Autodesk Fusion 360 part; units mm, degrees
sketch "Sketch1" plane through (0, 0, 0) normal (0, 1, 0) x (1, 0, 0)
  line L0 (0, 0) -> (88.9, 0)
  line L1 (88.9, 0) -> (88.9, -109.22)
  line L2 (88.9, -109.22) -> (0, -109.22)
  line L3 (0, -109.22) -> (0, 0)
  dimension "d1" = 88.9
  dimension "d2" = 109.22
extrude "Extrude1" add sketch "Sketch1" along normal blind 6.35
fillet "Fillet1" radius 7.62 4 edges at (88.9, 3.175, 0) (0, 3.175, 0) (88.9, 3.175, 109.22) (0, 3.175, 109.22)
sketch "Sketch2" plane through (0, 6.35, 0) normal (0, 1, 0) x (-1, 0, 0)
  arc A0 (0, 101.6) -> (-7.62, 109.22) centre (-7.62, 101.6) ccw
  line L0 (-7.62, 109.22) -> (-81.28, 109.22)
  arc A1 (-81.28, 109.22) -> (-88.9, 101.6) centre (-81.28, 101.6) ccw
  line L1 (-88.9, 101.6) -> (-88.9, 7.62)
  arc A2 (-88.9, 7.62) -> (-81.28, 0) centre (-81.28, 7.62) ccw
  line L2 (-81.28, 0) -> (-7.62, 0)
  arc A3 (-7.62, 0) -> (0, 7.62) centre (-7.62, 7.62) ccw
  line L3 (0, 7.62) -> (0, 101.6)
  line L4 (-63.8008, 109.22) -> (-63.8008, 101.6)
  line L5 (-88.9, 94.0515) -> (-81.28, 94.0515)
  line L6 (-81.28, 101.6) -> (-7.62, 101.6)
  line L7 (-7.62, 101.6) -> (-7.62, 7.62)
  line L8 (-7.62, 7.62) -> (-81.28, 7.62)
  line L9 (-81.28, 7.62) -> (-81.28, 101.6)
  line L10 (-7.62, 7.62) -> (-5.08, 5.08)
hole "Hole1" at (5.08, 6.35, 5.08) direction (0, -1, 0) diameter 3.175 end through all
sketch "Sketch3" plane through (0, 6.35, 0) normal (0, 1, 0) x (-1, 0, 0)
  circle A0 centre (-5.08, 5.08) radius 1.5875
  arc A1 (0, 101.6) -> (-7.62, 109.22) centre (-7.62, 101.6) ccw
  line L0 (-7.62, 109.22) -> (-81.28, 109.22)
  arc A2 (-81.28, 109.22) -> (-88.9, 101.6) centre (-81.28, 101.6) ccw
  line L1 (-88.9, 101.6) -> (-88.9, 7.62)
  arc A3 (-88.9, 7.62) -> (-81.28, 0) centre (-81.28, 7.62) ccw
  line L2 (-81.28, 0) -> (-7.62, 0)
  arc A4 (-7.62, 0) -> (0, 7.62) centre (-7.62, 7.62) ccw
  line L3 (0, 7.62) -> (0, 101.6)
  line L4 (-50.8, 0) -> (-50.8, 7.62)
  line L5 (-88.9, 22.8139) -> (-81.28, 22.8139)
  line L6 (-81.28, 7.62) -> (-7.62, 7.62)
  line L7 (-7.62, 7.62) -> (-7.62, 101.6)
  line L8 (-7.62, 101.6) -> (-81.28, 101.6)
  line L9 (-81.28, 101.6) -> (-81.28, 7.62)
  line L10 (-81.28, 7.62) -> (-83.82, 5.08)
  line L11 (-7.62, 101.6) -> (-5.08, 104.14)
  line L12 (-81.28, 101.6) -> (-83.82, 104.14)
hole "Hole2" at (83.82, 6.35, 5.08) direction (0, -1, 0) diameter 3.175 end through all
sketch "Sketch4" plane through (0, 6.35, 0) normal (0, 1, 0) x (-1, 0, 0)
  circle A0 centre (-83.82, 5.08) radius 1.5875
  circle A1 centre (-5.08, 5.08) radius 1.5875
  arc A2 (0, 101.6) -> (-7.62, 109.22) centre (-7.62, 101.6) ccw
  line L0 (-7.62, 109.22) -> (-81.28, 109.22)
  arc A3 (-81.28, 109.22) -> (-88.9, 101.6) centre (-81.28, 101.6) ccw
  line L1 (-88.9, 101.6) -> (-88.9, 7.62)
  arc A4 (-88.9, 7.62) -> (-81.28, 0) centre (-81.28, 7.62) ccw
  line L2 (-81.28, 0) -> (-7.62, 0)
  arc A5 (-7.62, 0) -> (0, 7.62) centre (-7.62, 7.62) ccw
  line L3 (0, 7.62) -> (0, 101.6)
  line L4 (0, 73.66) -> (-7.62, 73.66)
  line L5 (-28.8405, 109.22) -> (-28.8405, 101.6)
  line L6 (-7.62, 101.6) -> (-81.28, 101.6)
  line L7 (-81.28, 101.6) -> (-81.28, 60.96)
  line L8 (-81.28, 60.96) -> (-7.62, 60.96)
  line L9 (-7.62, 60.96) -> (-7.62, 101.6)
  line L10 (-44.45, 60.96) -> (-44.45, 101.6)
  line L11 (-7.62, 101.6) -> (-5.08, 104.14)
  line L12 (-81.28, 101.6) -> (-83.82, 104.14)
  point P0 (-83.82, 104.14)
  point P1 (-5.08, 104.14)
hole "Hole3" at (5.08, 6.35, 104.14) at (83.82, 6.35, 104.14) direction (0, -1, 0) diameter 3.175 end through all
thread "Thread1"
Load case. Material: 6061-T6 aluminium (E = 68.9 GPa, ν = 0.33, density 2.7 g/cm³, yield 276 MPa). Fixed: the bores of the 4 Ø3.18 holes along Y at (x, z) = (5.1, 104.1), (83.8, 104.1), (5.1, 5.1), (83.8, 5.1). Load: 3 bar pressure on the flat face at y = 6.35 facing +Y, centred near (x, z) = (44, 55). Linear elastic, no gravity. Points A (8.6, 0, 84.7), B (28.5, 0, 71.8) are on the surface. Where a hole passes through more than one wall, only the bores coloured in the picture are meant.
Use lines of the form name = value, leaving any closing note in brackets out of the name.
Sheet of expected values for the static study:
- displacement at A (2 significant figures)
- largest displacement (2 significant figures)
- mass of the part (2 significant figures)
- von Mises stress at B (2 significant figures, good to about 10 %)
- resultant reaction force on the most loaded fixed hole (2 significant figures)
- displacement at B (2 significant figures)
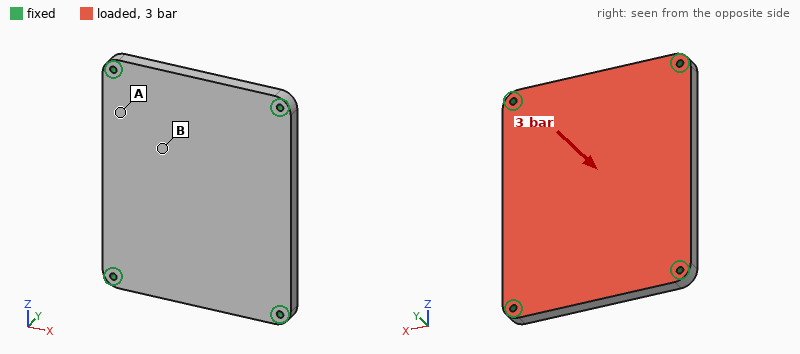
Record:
displacement at A = 0.051 mm
largest displacement = 0.12 mm
mass of the part = 170 g
von Mises stress at B = 19 MPa
resultant reaction force on the most loaded fixed hole = 720 N
displacement at B = 0.10 mm
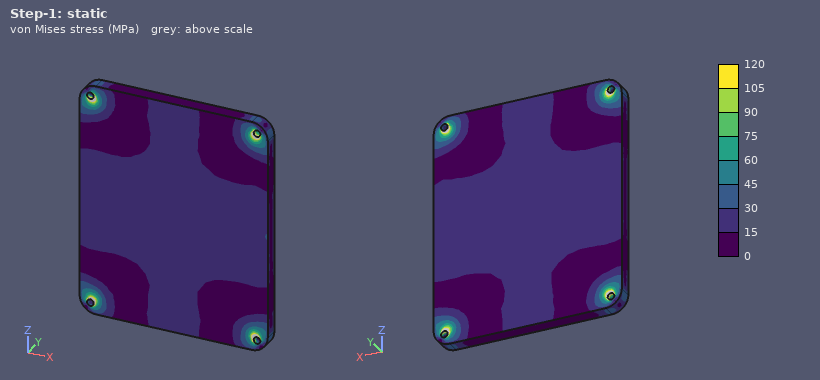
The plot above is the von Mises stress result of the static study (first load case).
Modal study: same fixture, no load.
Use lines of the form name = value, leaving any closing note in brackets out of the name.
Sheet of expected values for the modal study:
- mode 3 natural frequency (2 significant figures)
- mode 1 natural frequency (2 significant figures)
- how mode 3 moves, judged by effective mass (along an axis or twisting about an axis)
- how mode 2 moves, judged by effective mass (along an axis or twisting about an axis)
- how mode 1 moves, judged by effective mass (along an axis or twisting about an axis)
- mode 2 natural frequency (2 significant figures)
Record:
mode 3 natural frequency = 4700 Hz
mode 1 natural frequency = 2200 Hz
how mode 3 moves, judged by effective mass = twisting about X
how mode 2 moves, judged by effective mass = twisting about Z
how mode 1 moves, judged by effective mass = along Y
mode 2 natural frequency = 3700 Hz
